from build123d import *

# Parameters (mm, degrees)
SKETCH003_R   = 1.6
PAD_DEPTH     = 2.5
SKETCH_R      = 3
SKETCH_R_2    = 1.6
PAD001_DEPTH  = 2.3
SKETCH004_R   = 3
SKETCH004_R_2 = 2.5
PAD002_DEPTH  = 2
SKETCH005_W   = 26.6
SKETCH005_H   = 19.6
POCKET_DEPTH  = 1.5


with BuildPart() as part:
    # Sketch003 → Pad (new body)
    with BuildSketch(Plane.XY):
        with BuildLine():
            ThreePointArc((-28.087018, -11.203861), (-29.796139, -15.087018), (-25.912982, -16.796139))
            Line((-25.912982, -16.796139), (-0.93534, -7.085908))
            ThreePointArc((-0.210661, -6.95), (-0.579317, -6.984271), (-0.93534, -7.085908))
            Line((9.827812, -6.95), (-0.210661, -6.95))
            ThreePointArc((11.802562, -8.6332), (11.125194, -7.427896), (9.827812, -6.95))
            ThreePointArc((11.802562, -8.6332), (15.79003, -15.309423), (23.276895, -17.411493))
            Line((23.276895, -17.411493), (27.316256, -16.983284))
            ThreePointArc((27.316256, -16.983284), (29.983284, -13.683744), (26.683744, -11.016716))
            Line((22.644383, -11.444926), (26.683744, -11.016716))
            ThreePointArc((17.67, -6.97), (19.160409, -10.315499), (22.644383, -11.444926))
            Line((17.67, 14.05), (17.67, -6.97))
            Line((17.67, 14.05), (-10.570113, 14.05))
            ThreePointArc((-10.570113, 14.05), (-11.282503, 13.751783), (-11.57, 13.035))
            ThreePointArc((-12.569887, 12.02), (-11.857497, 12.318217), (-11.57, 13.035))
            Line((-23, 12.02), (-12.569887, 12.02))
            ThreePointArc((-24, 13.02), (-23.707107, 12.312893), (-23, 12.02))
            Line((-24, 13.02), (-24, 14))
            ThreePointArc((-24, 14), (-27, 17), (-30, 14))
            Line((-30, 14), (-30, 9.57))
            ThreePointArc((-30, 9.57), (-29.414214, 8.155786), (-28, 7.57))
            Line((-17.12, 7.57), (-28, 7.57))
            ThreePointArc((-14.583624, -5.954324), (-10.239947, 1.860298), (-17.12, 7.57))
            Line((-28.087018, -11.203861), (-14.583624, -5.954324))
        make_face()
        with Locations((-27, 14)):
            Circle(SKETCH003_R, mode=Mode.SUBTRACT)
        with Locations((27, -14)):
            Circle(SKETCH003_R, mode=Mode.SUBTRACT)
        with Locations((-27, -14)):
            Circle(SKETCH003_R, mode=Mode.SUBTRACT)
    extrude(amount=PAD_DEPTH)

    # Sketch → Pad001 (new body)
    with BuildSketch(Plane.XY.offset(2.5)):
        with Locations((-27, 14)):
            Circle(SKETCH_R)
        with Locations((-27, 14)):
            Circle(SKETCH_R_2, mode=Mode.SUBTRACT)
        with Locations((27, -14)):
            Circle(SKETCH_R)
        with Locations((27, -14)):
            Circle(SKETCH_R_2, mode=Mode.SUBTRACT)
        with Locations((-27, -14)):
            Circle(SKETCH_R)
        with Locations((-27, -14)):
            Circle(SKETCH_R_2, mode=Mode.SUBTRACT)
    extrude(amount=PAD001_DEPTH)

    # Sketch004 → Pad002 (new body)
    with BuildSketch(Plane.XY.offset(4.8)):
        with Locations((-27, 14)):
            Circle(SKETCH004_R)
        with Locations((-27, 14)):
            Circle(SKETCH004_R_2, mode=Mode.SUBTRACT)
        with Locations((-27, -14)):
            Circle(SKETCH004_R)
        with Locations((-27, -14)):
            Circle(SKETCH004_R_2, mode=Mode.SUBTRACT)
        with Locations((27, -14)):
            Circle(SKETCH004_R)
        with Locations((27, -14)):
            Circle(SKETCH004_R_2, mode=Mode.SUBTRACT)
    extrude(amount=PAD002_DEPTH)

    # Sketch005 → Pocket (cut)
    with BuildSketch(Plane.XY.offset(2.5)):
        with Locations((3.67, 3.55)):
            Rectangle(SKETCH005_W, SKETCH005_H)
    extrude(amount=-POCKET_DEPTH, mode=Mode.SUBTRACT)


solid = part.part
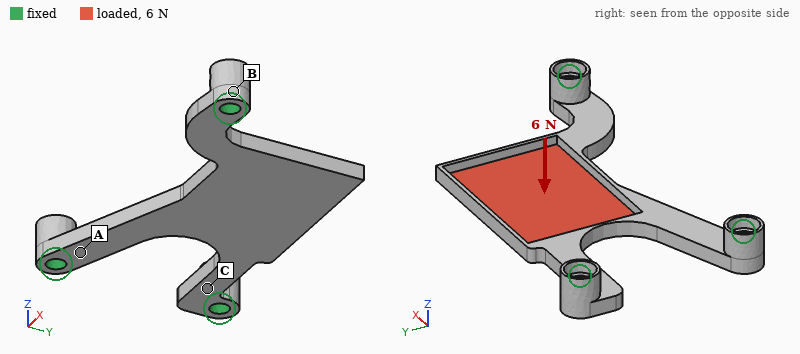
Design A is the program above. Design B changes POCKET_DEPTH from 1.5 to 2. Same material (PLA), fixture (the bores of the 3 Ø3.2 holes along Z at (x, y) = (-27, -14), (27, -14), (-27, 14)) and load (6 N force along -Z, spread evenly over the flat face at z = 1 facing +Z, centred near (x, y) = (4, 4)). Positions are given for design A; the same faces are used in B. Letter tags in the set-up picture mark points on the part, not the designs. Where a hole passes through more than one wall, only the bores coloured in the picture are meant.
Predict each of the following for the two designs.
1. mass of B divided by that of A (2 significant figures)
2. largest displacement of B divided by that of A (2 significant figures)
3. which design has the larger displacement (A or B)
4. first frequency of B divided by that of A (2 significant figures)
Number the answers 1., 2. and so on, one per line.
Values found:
1. 0.85
2. 1.2
3. B
4. 1.1
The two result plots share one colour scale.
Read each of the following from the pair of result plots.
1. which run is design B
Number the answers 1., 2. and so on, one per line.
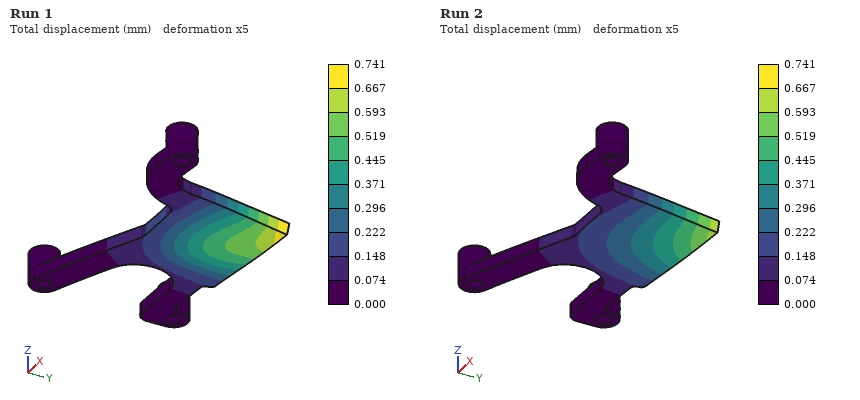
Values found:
1. Run 1
